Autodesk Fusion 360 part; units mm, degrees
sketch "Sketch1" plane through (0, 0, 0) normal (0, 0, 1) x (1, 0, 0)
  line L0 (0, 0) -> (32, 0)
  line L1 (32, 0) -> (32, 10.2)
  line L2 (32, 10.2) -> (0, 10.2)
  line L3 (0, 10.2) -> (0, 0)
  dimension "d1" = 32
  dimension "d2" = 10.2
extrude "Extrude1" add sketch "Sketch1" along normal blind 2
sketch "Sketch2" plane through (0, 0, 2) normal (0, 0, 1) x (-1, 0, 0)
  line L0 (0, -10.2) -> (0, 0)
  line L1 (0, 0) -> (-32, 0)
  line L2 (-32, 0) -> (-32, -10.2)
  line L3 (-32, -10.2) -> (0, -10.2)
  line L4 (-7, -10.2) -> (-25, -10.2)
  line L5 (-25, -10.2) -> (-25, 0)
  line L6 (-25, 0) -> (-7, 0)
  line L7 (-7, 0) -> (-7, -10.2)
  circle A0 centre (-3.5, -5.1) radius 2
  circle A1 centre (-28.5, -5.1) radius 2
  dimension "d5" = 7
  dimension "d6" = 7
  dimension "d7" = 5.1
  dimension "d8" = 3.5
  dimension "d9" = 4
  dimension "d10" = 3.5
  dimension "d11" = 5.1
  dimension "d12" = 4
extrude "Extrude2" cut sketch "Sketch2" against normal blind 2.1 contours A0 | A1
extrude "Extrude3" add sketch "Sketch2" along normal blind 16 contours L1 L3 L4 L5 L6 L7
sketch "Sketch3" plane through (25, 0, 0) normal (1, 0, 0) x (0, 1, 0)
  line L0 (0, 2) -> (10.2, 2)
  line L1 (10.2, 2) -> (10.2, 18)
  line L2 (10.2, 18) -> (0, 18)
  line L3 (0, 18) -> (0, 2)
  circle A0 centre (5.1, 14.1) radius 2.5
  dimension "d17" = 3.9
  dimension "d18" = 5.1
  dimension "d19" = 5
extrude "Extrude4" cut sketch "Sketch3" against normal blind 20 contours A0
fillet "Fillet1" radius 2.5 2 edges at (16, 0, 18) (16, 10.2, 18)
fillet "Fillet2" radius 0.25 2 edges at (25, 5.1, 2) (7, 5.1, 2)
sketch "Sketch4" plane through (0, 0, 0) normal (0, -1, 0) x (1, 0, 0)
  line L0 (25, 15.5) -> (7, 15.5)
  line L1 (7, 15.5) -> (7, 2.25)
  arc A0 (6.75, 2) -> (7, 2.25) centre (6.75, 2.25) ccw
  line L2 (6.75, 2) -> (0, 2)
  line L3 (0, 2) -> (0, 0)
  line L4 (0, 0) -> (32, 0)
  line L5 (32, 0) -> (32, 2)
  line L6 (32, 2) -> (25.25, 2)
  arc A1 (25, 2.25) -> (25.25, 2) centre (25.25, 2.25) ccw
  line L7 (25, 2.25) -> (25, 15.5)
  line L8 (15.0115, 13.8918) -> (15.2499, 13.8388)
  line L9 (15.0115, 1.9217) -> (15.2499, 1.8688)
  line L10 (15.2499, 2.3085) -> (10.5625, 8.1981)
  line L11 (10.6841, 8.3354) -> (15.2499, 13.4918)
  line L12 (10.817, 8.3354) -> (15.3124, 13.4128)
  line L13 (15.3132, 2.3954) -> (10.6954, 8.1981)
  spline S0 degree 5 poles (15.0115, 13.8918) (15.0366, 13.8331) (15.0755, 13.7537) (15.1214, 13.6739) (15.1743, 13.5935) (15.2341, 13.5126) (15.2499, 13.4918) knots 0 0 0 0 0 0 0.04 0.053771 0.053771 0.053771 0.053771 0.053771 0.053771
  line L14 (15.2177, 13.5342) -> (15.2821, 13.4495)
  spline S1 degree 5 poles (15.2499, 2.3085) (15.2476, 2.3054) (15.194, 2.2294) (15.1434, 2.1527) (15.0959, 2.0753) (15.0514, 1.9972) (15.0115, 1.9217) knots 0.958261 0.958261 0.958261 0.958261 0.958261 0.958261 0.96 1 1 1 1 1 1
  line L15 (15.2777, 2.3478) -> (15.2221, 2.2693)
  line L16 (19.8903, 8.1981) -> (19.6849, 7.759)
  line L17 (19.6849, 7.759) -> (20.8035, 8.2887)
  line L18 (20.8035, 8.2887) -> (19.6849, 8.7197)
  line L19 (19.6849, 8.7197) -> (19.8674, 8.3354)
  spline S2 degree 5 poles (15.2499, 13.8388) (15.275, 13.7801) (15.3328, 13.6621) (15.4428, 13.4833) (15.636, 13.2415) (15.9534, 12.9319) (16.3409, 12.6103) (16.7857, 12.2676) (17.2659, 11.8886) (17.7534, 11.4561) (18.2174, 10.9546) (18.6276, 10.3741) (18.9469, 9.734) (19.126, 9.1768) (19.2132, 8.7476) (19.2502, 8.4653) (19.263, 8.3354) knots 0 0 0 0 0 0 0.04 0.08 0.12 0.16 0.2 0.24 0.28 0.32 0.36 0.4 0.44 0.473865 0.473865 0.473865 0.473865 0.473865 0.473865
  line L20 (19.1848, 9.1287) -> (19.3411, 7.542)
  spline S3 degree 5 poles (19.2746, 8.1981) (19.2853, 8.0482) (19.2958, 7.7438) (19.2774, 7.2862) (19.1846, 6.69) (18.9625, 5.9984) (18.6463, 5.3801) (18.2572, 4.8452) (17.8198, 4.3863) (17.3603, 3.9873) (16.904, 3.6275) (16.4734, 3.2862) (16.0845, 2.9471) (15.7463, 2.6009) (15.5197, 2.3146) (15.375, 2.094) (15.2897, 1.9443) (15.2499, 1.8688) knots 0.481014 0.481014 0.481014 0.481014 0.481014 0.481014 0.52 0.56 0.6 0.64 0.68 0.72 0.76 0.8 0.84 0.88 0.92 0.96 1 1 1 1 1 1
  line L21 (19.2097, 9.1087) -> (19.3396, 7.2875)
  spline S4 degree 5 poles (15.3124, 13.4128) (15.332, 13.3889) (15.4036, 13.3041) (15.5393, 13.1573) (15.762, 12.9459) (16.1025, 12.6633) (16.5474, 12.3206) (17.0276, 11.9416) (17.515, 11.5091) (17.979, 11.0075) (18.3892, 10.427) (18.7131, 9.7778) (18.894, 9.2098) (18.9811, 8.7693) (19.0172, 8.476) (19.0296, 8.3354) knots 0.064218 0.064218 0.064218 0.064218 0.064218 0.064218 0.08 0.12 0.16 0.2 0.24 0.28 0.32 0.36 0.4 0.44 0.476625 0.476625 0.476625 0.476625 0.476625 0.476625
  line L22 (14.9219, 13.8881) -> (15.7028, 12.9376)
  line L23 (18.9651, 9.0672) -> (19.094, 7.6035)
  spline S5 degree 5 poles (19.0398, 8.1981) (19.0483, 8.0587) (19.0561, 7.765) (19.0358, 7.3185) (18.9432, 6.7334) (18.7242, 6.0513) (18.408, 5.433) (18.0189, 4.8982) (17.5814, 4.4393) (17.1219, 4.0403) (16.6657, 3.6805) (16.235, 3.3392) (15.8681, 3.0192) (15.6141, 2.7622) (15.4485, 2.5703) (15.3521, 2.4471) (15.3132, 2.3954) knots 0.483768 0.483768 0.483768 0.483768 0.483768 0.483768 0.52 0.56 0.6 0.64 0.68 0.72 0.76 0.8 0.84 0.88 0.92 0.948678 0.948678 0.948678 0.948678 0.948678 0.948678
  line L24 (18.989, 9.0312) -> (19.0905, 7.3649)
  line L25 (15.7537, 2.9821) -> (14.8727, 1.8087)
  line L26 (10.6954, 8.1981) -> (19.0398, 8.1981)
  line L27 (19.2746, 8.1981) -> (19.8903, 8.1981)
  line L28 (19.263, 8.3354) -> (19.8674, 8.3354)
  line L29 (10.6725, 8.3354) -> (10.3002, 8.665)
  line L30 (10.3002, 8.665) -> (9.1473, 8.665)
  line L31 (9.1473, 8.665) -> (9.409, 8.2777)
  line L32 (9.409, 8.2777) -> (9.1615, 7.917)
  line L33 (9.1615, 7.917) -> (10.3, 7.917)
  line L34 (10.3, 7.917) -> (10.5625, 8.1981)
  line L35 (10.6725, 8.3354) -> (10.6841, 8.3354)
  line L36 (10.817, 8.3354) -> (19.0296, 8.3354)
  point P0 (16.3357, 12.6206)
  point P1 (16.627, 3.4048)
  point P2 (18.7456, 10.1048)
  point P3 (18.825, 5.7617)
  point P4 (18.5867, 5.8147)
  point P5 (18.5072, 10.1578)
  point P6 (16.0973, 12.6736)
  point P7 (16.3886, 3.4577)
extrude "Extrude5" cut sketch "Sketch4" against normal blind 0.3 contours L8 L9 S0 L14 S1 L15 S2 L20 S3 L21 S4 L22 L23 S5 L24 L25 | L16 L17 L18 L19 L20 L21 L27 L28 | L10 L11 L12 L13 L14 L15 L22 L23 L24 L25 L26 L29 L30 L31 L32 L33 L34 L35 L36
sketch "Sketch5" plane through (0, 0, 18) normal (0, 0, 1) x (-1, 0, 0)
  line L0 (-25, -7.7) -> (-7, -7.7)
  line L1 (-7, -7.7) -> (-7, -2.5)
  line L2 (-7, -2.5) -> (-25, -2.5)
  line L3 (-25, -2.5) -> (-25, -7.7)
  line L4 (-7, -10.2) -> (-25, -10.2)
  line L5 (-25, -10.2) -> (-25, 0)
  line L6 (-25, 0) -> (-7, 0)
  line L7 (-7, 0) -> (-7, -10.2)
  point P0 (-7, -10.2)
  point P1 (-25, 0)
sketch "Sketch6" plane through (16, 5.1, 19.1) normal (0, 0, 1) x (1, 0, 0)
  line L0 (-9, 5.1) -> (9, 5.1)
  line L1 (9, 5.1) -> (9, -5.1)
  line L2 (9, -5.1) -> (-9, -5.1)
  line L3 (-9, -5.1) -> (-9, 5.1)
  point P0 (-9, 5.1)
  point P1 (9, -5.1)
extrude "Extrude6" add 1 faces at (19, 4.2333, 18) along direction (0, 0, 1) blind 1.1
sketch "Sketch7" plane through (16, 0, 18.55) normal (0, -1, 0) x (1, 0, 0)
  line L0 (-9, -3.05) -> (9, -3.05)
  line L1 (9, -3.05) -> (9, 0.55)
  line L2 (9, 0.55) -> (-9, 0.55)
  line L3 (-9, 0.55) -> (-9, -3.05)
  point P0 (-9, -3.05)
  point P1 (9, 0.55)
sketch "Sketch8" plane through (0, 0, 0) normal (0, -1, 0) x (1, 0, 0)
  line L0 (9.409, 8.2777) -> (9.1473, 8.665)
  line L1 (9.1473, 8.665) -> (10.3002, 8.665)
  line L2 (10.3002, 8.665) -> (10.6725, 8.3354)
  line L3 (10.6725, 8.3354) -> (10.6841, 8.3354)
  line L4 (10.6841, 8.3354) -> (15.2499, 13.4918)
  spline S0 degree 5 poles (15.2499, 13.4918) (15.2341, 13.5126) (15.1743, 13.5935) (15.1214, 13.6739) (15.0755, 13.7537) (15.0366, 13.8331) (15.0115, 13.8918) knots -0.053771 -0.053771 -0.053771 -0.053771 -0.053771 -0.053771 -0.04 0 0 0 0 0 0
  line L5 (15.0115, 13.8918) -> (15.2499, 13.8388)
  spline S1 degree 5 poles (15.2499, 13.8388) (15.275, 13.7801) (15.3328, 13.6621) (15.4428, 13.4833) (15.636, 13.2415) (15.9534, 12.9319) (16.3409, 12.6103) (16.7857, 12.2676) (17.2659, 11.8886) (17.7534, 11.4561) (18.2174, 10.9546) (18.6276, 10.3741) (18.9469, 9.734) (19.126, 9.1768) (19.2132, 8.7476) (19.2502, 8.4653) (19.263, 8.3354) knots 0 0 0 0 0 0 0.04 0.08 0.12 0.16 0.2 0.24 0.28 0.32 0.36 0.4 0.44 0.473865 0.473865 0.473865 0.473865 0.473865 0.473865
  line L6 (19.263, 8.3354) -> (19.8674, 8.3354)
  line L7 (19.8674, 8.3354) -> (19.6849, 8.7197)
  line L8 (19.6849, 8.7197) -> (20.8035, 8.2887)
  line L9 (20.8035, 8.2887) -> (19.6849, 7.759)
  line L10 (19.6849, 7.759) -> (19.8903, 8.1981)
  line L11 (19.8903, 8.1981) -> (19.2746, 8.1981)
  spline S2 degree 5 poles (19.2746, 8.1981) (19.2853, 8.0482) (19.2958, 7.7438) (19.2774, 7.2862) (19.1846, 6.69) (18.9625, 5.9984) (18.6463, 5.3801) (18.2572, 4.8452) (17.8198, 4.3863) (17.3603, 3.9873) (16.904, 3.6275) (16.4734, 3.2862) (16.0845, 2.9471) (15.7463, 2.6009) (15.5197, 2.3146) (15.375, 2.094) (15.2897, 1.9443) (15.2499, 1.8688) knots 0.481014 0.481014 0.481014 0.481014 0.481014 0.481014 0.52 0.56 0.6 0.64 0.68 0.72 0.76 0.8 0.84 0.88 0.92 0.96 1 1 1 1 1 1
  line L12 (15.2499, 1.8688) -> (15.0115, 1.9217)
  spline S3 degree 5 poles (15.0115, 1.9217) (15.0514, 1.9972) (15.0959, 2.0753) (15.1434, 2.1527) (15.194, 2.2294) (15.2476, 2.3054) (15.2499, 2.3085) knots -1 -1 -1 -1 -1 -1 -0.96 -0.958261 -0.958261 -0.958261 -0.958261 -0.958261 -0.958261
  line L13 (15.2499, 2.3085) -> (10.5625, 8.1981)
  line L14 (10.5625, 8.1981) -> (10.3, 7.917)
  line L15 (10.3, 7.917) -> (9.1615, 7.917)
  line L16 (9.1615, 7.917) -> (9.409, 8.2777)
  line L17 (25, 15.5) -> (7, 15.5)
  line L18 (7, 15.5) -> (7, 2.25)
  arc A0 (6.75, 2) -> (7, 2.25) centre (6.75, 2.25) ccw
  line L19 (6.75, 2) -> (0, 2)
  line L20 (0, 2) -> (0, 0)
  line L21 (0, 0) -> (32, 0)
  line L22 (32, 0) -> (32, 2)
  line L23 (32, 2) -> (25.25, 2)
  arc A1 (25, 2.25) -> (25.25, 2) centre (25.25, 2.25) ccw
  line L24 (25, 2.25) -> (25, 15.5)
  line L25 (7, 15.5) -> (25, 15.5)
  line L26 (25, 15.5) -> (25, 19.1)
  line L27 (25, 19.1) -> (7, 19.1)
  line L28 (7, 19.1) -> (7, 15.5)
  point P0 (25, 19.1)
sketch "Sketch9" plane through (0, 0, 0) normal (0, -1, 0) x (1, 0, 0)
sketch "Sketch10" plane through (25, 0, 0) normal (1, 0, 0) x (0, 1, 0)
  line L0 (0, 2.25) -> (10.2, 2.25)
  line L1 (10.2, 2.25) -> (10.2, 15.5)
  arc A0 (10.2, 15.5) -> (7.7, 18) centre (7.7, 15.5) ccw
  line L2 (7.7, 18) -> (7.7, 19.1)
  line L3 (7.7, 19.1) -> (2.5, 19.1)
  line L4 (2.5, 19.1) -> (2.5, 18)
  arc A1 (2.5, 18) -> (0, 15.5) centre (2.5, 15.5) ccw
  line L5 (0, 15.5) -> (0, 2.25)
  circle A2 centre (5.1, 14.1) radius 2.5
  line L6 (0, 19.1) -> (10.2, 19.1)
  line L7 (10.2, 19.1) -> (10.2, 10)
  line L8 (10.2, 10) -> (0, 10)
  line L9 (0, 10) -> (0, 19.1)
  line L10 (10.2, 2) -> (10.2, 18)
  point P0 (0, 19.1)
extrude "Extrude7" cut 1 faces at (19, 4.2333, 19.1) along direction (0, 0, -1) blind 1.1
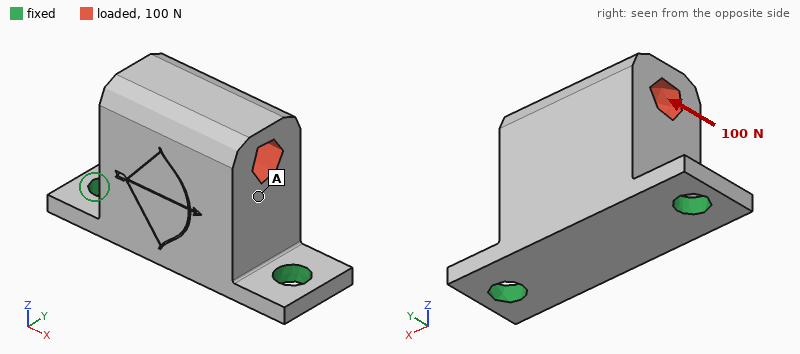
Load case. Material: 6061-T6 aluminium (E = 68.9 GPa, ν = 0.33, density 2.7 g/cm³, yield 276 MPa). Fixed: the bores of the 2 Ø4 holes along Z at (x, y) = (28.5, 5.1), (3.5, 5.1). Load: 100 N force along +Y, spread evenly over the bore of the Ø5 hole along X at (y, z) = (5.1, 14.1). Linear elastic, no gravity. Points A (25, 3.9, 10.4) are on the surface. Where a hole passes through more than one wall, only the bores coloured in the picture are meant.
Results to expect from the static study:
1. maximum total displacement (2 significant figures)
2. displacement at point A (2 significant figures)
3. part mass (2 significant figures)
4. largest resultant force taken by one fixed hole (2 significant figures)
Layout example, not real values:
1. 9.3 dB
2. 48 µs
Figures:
1. 30 µm
2. 17 µm
3. 8.5 g
4. 50 N
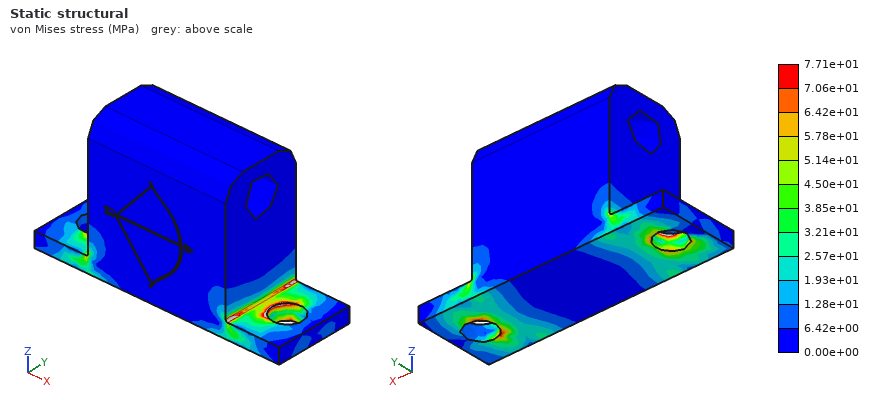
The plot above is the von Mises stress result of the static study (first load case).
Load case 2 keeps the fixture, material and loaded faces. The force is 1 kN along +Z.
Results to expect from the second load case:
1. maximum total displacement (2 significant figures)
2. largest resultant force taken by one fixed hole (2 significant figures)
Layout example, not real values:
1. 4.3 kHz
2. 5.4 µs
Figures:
1. 10.0 µm
2. 560 N
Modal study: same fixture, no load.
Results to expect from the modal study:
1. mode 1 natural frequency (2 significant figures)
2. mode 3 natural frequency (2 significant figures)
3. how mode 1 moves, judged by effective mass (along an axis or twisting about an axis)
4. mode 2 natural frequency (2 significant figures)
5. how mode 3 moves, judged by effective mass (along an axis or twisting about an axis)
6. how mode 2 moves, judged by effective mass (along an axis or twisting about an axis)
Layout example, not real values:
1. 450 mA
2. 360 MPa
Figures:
1. 5200 Hz
2. 20 kHz
3. along Y
4. 18 kHz
5. along Z
6. along X
